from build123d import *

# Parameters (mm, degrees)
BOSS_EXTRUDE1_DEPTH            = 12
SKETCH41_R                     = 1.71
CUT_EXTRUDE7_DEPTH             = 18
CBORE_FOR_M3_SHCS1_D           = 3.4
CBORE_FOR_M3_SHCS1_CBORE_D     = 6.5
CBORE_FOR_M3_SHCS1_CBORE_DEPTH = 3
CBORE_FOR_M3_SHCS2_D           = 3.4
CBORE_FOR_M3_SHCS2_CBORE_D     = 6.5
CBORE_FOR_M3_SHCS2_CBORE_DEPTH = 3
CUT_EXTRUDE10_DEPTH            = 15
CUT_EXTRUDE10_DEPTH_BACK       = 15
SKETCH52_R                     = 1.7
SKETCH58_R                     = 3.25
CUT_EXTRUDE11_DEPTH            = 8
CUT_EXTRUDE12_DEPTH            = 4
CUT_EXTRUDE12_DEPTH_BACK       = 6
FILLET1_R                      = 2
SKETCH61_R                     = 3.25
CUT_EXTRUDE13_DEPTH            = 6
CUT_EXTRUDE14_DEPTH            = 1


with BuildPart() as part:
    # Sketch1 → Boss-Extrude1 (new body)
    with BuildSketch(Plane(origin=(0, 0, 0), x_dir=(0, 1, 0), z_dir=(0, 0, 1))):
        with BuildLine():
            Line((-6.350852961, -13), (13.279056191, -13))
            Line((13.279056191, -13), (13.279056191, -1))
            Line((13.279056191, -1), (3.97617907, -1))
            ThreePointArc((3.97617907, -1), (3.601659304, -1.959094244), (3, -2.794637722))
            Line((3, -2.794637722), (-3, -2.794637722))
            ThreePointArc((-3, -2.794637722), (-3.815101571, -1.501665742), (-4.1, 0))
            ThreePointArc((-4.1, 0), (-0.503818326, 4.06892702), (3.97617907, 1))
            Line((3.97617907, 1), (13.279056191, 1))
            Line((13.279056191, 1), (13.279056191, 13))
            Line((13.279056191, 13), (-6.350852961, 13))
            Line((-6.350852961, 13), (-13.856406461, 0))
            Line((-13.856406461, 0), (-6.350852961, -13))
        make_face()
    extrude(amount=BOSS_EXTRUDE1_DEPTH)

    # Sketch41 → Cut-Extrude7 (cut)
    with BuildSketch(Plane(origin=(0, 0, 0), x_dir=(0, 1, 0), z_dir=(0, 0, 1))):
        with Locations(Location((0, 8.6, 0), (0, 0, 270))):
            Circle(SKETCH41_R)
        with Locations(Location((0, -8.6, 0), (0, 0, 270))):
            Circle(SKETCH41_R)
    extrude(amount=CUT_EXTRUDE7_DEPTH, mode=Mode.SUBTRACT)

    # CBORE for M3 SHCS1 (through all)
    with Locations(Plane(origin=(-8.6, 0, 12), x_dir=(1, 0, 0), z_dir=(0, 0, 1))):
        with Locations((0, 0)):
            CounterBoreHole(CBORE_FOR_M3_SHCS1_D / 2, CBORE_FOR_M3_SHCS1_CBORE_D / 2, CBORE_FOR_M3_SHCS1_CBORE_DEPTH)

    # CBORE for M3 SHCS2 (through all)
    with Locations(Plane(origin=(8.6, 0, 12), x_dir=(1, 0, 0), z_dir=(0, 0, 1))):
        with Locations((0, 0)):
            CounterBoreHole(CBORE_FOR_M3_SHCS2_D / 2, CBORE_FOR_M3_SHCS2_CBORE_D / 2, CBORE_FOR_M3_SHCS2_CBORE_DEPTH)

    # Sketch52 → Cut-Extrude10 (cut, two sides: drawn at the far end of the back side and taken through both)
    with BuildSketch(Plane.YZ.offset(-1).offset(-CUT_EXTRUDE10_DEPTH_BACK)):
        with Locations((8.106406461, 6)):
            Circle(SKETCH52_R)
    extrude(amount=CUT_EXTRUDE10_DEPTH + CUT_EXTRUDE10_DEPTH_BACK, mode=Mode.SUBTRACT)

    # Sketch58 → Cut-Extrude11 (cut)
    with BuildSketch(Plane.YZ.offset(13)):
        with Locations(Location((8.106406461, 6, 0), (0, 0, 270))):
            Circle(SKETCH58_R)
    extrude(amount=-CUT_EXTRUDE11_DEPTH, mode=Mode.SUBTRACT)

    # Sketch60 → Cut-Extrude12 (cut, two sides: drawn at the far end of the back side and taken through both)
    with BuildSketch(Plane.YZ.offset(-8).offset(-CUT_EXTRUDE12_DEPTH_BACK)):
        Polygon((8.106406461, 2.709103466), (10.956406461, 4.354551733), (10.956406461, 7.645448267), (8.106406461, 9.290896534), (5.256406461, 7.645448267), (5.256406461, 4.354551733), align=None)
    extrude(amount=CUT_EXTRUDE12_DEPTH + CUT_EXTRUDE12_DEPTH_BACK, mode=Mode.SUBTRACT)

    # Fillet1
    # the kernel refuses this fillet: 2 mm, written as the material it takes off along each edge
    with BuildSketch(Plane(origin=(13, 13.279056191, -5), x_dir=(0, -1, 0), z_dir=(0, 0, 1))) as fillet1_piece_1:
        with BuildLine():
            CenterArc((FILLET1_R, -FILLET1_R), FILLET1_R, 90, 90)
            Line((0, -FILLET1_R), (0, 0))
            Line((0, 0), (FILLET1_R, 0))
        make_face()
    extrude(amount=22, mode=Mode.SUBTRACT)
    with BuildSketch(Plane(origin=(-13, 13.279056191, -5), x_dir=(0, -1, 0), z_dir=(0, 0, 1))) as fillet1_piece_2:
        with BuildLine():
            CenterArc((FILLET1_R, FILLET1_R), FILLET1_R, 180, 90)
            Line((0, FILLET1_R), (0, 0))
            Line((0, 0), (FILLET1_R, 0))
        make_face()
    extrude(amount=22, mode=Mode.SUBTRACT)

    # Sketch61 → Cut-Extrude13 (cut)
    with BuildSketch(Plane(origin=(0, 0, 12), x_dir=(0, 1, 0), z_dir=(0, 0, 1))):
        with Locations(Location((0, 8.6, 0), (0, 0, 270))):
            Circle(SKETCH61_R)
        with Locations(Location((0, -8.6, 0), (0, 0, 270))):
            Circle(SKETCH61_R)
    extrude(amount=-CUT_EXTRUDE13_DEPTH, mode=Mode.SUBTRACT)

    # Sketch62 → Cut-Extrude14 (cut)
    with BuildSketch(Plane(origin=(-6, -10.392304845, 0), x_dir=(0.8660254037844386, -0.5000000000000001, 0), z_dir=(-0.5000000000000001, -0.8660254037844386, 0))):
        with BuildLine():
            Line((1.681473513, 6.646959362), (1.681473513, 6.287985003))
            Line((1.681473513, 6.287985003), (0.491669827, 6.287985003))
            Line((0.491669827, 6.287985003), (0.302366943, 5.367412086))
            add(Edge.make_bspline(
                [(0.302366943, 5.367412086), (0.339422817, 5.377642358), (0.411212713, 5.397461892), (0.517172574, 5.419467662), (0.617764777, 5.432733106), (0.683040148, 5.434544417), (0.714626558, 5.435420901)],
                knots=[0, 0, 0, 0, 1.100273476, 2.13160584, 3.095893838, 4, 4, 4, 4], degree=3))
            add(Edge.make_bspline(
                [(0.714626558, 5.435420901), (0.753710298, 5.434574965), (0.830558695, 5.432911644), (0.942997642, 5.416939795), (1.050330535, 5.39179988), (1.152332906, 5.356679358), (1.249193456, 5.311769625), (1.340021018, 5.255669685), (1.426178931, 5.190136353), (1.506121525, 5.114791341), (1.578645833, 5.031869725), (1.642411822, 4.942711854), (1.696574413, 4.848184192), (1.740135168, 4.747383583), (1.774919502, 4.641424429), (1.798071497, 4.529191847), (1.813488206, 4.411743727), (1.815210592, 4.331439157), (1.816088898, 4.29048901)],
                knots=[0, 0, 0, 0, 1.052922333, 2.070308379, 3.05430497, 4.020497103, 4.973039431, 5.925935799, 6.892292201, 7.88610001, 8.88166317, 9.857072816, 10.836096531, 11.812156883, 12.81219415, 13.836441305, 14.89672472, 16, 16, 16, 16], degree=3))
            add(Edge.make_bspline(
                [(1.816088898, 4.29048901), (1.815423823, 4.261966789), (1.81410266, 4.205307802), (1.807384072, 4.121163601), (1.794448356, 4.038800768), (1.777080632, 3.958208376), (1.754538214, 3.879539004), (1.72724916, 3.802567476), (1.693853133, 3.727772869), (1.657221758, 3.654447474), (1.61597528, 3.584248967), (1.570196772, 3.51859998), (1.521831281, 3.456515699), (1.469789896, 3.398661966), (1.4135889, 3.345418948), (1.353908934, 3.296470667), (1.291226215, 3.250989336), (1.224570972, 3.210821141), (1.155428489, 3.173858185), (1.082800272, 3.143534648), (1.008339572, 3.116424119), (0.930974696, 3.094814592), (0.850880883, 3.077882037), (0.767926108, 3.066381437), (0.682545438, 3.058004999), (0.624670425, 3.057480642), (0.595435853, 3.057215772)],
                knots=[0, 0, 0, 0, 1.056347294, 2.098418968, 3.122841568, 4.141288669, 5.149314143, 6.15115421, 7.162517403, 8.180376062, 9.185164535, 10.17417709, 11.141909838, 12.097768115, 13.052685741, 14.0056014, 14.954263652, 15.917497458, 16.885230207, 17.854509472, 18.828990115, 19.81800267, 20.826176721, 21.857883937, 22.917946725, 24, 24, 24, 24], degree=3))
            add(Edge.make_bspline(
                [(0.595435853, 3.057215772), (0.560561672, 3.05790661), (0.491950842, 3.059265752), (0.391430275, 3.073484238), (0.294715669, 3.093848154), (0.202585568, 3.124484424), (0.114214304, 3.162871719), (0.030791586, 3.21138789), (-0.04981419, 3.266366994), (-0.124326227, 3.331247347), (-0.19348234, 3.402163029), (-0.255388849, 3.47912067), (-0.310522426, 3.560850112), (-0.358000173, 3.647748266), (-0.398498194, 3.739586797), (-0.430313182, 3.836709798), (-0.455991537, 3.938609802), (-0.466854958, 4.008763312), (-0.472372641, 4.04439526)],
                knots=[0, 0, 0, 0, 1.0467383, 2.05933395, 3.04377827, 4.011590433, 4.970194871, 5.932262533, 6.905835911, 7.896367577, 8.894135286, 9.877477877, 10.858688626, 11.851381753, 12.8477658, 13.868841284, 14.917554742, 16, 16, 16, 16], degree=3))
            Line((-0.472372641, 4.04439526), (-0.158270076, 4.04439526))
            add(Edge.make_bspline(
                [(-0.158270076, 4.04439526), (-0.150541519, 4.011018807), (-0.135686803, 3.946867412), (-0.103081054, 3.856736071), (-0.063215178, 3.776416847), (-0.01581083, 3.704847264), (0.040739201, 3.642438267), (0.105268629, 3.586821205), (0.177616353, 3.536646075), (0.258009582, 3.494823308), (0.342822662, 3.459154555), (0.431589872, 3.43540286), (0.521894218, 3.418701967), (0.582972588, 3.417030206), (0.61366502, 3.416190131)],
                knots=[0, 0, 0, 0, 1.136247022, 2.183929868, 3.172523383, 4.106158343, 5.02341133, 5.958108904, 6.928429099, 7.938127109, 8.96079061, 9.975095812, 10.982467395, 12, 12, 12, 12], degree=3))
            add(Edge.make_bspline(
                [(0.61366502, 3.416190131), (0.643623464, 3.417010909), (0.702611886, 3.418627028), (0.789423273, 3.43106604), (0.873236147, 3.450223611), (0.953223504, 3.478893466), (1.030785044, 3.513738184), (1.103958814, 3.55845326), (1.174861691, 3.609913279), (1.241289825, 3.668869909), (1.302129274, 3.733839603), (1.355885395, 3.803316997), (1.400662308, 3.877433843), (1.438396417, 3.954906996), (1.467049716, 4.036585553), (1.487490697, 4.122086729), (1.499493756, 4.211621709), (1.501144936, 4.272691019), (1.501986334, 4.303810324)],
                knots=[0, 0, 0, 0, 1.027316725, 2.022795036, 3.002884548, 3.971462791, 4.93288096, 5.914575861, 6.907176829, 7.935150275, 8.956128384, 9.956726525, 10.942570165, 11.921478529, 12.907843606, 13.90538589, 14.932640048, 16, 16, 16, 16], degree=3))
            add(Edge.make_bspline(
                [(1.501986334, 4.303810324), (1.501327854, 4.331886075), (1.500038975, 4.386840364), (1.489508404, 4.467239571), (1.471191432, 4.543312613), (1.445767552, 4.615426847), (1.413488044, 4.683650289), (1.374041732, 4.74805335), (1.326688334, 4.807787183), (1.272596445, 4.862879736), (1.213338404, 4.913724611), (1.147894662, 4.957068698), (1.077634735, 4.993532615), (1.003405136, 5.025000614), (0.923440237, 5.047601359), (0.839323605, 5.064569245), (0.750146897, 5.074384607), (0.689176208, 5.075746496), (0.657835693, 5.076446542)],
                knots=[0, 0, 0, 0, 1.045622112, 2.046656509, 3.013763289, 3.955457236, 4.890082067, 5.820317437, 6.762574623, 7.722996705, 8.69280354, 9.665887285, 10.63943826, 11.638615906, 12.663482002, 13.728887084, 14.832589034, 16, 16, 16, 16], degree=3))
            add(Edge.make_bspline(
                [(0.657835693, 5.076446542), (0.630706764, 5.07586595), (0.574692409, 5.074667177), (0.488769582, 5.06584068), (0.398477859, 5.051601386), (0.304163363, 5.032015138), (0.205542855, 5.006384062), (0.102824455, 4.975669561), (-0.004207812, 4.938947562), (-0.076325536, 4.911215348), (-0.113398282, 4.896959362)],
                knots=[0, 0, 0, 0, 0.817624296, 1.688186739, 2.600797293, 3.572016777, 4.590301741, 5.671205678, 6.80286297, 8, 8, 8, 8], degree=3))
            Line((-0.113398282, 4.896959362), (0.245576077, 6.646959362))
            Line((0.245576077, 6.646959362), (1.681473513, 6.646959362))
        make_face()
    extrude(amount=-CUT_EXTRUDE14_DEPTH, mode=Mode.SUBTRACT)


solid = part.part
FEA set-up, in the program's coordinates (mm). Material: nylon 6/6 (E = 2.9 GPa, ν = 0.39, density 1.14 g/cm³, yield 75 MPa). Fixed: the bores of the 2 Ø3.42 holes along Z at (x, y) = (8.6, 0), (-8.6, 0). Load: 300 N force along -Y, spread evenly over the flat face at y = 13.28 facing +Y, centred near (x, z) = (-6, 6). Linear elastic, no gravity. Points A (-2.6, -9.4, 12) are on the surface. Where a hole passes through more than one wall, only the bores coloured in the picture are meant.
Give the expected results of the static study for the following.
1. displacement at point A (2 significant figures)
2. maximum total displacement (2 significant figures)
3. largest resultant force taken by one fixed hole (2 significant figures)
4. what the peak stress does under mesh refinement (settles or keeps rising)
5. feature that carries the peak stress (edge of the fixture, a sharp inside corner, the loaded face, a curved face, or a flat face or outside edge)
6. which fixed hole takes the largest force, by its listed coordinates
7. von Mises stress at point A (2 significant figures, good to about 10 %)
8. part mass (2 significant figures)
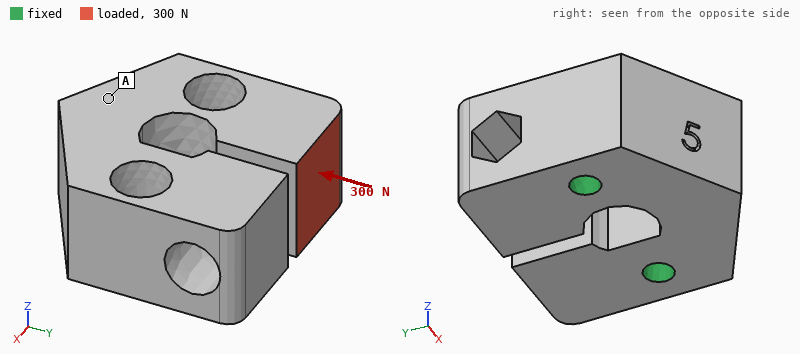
28 µm
89 µm
270 N
keeps rising
edge of the fixture
(-8.6, 0)
1.7 MPa
6.1 g
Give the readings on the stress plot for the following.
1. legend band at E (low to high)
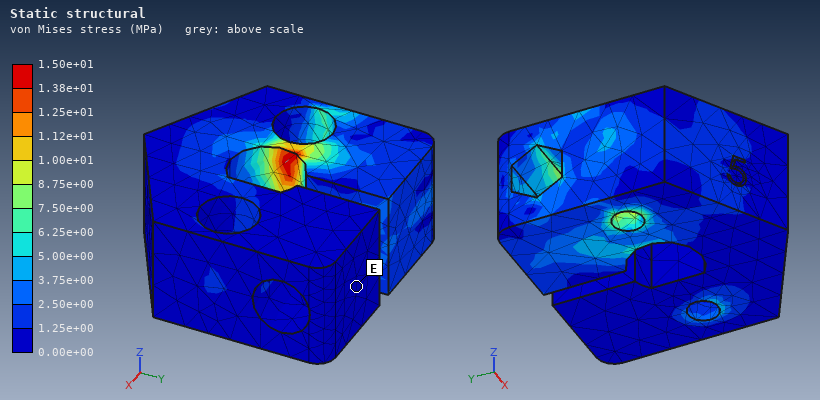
0.00e+00 to 1.25e+00 MPa
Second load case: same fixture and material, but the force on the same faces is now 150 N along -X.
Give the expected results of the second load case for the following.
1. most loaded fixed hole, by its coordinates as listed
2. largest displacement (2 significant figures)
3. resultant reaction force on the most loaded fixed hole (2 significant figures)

(-8.6, 0)
0.17 mm
210 N
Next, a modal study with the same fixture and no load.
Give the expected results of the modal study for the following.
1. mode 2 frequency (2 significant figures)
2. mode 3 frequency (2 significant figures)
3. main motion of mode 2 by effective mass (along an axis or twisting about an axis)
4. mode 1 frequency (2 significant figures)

6100 Hz
6400 Hz
along X
5400 Hz
